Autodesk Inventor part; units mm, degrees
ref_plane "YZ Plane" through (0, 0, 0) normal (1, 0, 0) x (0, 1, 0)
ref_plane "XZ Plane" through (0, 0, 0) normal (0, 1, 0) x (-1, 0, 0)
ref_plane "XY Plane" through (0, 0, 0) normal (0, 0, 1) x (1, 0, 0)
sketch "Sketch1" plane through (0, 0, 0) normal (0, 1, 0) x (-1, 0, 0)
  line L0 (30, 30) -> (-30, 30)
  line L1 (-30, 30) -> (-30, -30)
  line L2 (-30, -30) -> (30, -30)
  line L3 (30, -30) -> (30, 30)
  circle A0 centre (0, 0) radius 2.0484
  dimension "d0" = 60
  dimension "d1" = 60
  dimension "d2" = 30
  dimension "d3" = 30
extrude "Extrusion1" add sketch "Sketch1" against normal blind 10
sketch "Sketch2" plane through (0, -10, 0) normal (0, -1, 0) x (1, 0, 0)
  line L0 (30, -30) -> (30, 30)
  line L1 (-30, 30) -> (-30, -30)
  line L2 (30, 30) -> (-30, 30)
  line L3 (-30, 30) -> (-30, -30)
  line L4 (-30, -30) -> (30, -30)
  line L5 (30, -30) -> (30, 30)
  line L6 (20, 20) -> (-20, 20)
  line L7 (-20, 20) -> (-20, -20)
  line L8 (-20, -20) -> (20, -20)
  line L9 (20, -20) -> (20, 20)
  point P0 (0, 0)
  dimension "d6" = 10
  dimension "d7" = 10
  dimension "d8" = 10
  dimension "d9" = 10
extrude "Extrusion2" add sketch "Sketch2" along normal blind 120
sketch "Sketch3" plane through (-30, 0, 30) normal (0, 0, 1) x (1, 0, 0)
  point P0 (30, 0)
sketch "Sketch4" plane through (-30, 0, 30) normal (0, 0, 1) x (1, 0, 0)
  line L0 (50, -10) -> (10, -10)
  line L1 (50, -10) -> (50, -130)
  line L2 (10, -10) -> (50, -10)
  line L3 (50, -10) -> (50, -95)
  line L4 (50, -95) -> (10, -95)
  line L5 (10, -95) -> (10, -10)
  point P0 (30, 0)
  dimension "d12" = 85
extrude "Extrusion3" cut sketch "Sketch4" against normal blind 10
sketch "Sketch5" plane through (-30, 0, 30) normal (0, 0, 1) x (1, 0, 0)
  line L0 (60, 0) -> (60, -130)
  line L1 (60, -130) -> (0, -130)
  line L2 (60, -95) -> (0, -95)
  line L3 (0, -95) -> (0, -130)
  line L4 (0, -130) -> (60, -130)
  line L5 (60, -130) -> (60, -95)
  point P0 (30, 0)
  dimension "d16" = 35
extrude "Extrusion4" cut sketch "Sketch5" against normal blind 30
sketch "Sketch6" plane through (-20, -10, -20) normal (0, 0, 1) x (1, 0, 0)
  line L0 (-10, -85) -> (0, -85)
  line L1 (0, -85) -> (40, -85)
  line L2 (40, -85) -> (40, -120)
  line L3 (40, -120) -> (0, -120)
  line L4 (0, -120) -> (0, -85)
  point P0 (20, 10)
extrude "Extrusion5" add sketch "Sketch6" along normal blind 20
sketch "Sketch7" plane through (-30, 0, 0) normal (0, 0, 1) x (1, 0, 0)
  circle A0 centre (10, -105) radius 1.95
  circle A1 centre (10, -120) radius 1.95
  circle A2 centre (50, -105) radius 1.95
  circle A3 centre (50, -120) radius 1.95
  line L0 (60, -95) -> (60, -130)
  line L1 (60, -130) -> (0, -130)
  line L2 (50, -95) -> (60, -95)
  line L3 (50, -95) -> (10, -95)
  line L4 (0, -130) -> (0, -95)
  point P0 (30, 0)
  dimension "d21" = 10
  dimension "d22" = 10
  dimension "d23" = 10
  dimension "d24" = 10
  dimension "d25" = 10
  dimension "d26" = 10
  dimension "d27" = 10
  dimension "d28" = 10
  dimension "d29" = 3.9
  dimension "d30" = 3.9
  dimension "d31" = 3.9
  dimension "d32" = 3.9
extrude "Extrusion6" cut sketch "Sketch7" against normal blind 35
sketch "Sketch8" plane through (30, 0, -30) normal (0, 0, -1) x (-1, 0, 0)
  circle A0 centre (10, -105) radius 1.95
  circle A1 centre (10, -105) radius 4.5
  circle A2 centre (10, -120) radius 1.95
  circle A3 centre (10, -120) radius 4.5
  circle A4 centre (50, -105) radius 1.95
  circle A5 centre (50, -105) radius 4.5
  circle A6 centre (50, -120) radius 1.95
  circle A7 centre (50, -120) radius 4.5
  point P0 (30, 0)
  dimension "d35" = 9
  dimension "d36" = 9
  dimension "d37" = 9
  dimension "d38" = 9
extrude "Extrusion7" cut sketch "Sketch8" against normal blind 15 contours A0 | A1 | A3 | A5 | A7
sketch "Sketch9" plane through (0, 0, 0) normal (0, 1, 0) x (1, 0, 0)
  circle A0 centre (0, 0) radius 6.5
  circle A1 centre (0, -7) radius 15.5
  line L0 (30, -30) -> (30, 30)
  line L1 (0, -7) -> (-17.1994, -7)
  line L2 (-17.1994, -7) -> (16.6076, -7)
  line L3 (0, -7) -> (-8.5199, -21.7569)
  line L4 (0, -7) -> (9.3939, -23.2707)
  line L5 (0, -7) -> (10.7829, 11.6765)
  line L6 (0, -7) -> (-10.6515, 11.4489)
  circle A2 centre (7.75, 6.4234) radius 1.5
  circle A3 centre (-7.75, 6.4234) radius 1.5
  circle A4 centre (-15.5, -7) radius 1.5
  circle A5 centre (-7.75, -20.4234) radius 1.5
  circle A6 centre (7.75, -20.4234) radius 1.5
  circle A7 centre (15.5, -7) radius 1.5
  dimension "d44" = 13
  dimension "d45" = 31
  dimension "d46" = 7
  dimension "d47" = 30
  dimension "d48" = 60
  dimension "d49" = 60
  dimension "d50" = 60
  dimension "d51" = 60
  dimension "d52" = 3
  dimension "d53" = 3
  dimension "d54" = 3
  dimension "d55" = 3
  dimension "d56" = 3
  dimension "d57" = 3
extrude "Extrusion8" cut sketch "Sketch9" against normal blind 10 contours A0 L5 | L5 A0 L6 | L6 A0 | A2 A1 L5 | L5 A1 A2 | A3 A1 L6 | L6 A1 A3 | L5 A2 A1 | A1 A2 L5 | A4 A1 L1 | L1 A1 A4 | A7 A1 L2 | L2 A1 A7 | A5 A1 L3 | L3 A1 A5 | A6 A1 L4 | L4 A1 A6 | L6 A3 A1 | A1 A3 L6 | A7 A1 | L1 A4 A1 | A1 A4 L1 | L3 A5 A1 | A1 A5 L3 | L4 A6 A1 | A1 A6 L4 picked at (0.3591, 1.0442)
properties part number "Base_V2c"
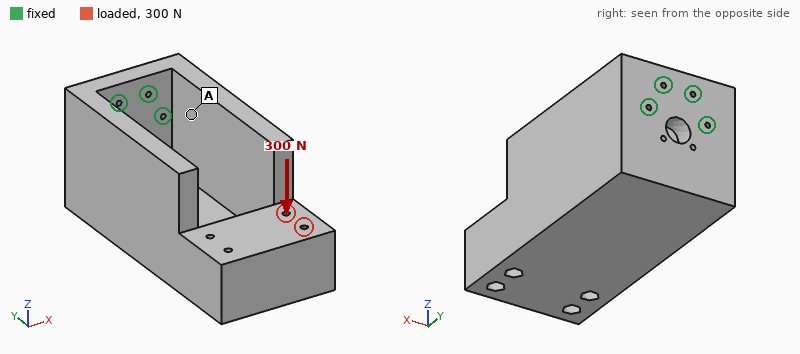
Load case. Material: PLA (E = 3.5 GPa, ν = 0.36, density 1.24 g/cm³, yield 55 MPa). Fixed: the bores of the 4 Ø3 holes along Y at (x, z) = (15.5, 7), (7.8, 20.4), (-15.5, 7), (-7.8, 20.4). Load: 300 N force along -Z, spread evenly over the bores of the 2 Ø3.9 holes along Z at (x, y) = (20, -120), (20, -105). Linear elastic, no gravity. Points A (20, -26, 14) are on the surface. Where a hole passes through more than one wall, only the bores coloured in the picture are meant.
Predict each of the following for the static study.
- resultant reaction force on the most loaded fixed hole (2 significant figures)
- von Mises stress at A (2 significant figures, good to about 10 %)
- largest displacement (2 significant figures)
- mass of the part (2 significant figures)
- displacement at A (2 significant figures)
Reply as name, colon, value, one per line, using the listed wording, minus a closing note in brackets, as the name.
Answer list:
resultant reaction force on the most loaded fixed hole: 650 N
von Mises stress at A: 3.5 MPa
largest displacement: 1.5 mm
mass of the part: 280 g
displacement at A: 0.24 mm
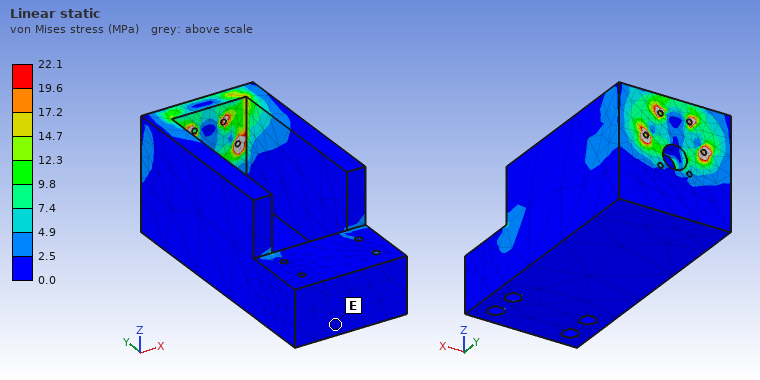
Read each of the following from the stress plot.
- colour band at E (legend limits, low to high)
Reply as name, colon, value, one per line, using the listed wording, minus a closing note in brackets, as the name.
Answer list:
colour band at E: 0.0 to 2.5 MPa
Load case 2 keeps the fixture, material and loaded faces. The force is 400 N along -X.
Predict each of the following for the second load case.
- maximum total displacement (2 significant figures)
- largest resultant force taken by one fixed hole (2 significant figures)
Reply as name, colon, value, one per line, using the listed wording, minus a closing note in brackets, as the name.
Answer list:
maximum total displacement: 1.4 mm
largest resultant force taken by one fixed hole: 1.0 kN
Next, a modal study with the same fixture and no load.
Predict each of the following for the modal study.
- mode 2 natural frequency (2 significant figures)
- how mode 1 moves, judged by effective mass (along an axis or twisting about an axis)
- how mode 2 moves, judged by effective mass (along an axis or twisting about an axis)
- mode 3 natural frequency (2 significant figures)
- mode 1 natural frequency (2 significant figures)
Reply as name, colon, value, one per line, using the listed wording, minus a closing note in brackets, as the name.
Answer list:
mode 2 natural frequency: 270 Hz
how mode 1 moves, judged by effective mass: along Z
how mode 2 moves, judged by effective mass: along X
mode 3 natural frequency: 950 Hz
mode 1 natural frequency: 230 Hz
